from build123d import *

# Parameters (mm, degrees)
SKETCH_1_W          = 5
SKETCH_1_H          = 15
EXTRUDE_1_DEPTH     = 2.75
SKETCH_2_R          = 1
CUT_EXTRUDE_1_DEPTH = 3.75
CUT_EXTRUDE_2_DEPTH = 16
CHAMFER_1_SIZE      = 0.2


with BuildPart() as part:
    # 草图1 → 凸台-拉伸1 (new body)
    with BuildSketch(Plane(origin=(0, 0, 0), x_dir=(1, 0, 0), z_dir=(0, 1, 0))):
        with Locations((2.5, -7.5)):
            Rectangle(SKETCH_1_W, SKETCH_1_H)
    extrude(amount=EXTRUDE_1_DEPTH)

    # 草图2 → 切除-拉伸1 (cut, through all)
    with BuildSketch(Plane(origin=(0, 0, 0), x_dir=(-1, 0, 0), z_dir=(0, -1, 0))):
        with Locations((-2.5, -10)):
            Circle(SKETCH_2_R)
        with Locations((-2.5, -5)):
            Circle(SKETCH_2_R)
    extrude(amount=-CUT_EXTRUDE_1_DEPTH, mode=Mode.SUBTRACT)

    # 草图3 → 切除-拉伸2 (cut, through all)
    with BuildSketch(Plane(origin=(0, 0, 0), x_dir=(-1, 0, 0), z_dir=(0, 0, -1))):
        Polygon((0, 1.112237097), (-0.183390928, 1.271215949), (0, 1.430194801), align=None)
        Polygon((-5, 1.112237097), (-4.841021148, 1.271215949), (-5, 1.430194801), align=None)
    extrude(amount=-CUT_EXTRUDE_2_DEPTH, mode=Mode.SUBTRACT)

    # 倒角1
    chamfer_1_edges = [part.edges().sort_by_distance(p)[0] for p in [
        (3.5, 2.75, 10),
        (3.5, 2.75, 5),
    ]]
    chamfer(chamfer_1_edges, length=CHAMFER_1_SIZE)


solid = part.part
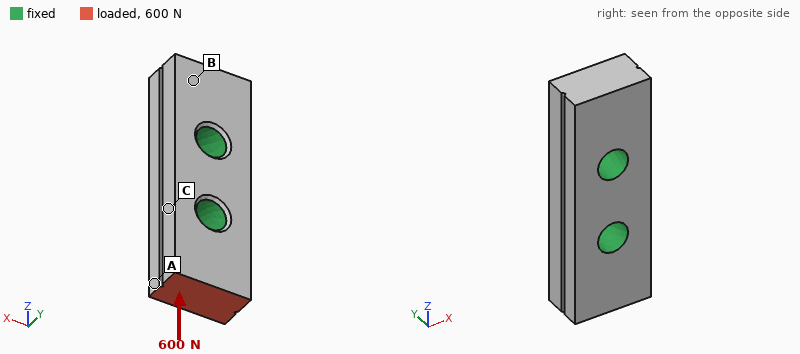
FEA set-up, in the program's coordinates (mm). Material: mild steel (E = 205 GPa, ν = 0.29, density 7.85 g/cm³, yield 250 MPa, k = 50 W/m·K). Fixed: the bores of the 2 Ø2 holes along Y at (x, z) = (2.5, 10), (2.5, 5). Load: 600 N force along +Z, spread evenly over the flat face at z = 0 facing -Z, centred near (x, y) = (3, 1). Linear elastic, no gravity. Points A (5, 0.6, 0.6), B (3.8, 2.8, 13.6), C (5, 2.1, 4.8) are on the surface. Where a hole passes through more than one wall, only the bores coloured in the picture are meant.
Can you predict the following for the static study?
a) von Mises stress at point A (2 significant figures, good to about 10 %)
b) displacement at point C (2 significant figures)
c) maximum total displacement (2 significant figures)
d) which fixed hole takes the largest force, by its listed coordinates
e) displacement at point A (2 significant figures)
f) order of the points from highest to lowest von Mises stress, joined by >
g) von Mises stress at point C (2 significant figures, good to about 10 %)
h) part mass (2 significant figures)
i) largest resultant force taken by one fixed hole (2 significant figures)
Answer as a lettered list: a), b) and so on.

a) 44 MPa
b) 0.28 µm
c) 1.1 µm
d) (2.5, 5)
e) 0.94 µm
f) A > C > B
g) 24 MPa
h) 1.5 g
i) 550 N
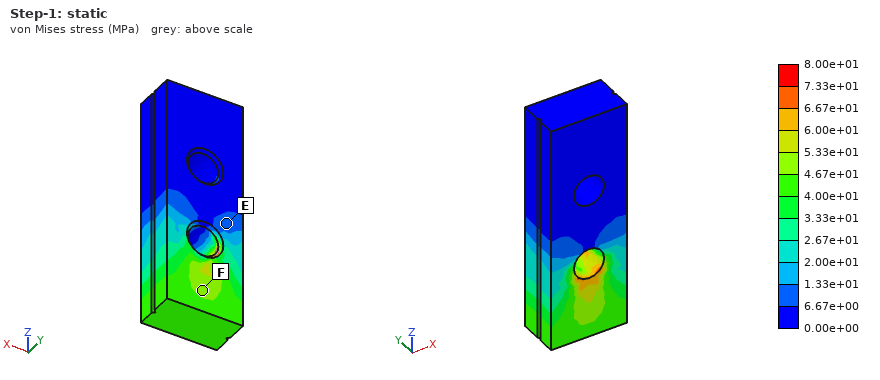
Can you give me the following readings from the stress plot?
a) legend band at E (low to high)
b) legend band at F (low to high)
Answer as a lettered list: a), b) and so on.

a) 6.67e+00 to 1.33e+01 MPa
b) 4.67e+01 to 5.33e+01 MPa
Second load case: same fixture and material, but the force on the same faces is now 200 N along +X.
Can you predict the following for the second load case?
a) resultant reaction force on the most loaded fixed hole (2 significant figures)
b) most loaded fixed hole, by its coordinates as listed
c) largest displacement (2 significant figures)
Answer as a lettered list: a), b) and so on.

a) 260 N
b) (2.5, 5)
c) 3.5 µm
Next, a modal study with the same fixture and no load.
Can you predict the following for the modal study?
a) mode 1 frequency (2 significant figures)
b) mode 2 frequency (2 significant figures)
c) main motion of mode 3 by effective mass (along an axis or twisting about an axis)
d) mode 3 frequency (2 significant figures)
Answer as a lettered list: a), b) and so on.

a) 87 kHz
b) 87 kHz
c) twisting about Y
d) 97 kHz
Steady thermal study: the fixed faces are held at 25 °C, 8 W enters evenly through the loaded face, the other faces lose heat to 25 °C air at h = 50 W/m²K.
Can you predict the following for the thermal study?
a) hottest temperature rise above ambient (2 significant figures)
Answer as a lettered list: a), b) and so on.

a) 53 K
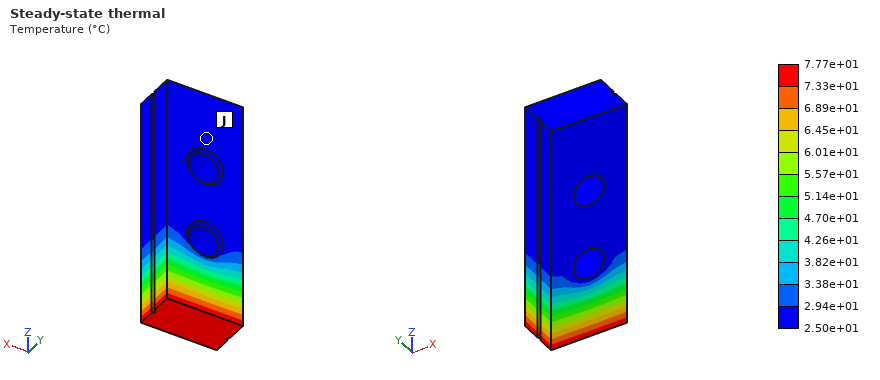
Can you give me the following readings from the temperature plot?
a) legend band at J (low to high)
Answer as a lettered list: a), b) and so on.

a) 2.50e+01 to 2.94e+01 °C
